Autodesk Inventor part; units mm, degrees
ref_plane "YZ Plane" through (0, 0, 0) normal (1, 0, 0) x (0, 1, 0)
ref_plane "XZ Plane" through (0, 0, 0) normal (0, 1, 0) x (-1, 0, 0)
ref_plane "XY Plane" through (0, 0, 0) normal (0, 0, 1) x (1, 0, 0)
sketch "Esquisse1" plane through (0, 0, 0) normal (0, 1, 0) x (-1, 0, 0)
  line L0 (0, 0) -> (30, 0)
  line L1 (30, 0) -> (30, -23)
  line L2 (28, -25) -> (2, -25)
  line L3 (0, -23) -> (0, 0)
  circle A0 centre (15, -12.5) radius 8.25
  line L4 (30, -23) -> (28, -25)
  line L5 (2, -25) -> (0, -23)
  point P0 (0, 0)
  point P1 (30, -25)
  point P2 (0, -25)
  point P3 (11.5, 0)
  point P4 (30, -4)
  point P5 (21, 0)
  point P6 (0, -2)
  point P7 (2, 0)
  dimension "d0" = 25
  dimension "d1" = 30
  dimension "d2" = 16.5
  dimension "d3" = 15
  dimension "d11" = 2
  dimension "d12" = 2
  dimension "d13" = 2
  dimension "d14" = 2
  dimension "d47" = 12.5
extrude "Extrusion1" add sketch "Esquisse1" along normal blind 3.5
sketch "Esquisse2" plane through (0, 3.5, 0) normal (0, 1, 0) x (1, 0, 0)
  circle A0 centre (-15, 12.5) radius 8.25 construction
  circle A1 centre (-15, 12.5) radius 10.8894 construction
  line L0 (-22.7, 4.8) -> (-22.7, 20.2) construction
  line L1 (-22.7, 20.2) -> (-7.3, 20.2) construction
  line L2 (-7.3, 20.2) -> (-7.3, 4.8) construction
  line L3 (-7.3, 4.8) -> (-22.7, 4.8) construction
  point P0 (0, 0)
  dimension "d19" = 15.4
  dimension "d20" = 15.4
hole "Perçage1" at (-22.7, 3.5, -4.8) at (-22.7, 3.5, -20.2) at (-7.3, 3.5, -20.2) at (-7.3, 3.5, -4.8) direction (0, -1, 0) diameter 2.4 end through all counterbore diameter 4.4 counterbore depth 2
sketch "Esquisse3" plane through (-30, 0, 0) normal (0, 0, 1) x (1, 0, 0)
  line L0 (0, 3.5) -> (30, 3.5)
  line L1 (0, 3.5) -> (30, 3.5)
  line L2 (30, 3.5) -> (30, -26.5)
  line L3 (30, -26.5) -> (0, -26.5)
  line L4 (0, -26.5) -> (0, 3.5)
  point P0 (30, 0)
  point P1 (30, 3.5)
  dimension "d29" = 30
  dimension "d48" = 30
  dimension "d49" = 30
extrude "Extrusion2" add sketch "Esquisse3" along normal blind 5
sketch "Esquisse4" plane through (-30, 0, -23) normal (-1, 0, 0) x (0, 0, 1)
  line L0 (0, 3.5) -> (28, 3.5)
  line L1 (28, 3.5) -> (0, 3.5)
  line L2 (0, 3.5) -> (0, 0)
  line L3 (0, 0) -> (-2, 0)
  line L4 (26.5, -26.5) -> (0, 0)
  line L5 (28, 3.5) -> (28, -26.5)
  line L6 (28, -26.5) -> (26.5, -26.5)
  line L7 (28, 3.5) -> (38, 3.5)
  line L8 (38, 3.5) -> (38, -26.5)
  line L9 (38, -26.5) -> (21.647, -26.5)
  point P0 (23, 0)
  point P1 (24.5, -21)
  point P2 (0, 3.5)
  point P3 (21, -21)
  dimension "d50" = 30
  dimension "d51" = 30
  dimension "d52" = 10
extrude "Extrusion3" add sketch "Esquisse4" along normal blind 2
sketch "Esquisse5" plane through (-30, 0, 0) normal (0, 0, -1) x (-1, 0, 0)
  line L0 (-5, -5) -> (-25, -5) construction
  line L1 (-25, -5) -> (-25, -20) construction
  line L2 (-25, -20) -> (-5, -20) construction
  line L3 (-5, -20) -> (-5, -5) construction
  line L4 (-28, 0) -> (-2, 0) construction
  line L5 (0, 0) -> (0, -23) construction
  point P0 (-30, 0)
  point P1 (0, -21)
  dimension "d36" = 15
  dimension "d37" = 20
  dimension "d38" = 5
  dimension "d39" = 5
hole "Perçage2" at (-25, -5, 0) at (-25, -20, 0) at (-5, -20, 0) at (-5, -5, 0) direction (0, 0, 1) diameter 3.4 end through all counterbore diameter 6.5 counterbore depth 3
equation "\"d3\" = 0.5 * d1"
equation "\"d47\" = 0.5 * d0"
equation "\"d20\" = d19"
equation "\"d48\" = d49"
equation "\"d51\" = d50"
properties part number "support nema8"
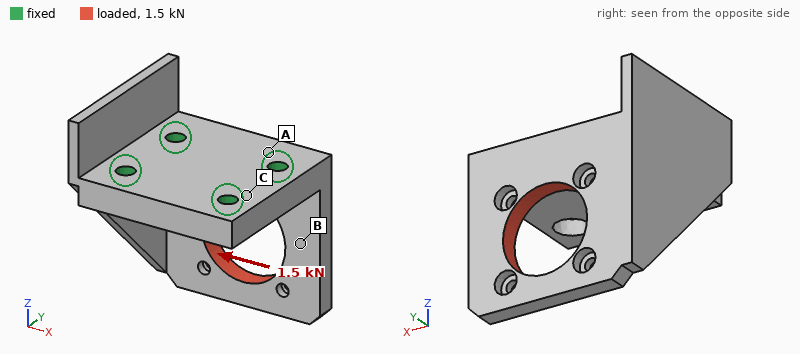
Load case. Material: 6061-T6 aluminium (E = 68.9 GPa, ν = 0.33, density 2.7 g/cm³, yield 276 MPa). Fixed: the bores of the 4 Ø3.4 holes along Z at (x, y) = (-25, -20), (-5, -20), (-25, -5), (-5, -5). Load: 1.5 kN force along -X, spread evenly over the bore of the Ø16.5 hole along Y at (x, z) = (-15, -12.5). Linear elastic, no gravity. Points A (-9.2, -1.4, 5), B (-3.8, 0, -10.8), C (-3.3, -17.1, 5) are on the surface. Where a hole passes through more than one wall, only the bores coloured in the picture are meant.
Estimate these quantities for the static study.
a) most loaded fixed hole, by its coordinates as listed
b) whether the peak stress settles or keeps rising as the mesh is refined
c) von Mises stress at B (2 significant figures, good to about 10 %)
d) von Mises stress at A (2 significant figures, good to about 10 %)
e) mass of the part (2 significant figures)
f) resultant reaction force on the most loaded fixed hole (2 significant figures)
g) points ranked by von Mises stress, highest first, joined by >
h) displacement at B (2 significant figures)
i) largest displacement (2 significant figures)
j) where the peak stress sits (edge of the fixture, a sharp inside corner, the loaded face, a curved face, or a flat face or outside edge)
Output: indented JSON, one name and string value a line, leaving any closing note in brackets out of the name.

{
  "most loaded fixed hole, by its coordinates as listed": "(-5, -5)",
  "whether the peak stress settles or keeps rising as the mesh is refined": "keeps rising",
  "von Mises stress at B": "60 MPa",
  "von Mises stress at A": "31 MPa",
  "mass of the part": "20 g",
  "resultant reaction force on the most loaded fixed hole": "1.5 kN",
  "points ranked by von Mises stress, highest first, joined by >": "B > A > C",
  "displacement at B": "0.062 mm",
  "largest displacement": "0.11 mm",
  "where the peak stress sits": "edge of the fixture"
}
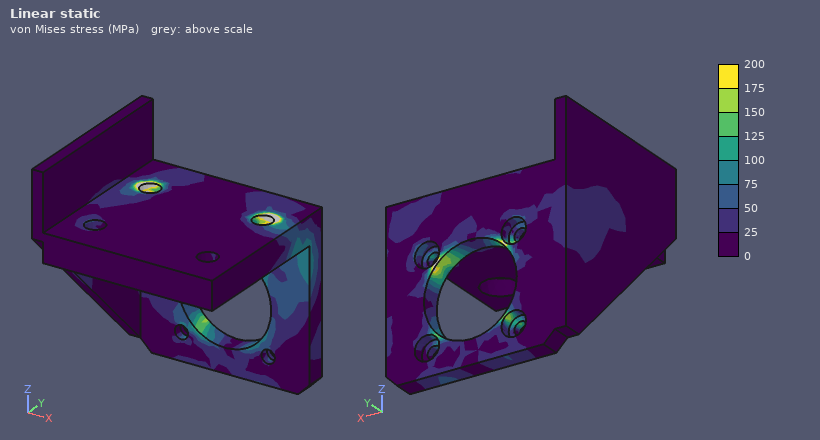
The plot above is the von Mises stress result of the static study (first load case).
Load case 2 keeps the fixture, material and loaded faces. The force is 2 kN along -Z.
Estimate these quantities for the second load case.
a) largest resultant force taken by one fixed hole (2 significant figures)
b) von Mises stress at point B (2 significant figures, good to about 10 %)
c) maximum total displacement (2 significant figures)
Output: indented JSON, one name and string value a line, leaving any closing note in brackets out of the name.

{
  "largest resultant force taken by one fixed hole": "1.4 kN",
  "von Mises stress at point B": "48 MPa",
  "maximum total displacement": "0.11 mm"
}
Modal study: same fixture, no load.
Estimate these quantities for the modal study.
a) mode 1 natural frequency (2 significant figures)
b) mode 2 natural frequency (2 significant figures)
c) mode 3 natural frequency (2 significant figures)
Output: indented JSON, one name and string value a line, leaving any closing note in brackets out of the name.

{
  "mode 1 natural frequency": "4400 Hz",
  "mode 2 natural frequency": "8100 Hz",
  "mode 3 natural frequency": "11 kHz"
}
